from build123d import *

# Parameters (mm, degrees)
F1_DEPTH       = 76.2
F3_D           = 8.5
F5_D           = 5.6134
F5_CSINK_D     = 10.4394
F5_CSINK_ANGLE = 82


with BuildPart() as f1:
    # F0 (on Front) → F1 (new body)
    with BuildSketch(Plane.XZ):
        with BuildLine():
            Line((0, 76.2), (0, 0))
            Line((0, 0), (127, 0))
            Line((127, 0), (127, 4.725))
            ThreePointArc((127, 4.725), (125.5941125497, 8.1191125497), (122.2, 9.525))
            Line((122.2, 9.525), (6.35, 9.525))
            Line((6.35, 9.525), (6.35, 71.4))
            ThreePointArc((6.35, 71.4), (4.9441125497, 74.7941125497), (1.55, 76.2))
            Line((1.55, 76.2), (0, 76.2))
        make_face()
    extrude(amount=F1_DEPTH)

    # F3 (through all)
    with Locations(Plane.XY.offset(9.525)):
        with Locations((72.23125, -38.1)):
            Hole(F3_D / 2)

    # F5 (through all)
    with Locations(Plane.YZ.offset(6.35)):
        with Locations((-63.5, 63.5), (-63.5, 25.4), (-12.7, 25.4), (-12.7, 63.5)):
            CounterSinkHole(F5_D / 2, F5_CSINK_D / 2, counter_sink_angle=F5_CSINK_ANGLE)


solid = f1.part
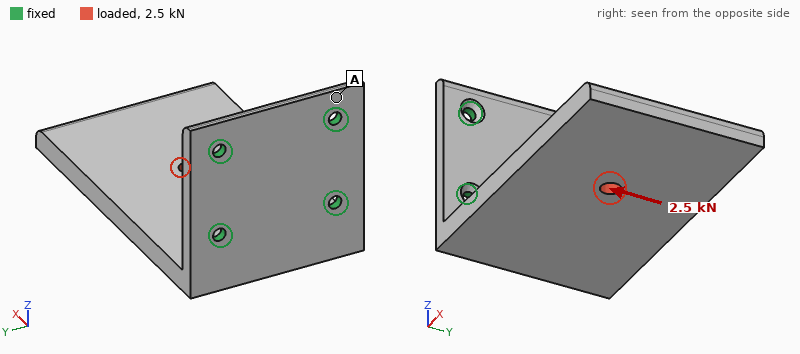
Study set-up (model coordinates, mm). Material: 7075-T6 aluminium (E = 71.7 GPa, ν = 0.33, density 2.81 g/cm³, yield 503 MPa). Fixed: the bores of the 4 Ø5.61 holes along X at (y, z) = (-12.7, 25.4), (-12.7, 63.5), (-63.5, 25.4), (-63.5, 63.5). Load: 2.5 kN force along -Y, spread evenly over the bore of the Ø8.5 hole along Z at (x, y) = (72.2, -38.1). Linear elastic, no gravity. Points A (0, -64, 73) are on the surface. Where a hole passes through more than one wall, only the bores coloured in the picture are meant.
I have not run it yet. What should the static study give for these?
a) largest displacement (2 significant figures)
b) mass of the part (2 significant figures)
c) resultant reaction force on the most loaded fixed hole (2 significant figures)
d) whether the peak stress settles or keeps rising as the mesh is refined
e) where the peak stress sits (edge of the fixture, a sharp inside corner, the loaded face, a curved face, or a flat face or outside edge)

0.56 mm
340 g
4.0 kN
keeps rising
edge of the fixture
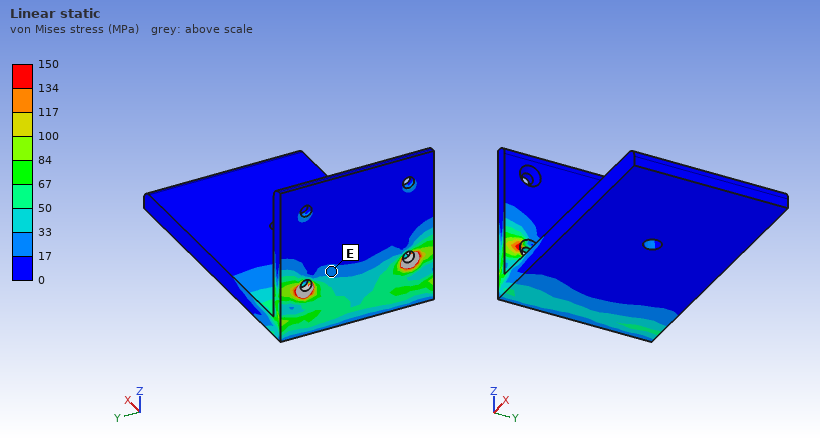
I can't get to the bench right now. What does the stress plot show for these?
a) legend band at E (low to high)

17 to 33 MPa
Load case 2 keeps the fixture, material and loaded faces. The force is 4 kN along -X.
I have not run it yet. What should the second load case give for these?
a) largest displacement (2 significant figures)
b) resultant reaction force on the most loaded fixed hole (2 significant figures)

1.3 mm
2.8 kN
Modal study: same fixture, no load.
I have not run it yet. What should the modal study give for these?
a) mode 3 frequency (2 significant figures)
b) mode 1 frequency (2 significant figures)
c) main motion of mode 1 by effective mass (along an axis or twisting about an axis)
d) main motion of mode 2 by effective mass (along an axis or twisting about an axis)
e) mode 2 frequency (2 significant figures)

1700 Hz
280 Hz
along Z
along Y
850 Hz
